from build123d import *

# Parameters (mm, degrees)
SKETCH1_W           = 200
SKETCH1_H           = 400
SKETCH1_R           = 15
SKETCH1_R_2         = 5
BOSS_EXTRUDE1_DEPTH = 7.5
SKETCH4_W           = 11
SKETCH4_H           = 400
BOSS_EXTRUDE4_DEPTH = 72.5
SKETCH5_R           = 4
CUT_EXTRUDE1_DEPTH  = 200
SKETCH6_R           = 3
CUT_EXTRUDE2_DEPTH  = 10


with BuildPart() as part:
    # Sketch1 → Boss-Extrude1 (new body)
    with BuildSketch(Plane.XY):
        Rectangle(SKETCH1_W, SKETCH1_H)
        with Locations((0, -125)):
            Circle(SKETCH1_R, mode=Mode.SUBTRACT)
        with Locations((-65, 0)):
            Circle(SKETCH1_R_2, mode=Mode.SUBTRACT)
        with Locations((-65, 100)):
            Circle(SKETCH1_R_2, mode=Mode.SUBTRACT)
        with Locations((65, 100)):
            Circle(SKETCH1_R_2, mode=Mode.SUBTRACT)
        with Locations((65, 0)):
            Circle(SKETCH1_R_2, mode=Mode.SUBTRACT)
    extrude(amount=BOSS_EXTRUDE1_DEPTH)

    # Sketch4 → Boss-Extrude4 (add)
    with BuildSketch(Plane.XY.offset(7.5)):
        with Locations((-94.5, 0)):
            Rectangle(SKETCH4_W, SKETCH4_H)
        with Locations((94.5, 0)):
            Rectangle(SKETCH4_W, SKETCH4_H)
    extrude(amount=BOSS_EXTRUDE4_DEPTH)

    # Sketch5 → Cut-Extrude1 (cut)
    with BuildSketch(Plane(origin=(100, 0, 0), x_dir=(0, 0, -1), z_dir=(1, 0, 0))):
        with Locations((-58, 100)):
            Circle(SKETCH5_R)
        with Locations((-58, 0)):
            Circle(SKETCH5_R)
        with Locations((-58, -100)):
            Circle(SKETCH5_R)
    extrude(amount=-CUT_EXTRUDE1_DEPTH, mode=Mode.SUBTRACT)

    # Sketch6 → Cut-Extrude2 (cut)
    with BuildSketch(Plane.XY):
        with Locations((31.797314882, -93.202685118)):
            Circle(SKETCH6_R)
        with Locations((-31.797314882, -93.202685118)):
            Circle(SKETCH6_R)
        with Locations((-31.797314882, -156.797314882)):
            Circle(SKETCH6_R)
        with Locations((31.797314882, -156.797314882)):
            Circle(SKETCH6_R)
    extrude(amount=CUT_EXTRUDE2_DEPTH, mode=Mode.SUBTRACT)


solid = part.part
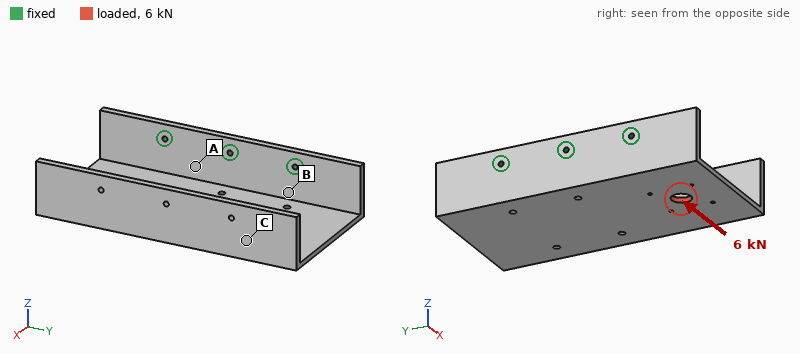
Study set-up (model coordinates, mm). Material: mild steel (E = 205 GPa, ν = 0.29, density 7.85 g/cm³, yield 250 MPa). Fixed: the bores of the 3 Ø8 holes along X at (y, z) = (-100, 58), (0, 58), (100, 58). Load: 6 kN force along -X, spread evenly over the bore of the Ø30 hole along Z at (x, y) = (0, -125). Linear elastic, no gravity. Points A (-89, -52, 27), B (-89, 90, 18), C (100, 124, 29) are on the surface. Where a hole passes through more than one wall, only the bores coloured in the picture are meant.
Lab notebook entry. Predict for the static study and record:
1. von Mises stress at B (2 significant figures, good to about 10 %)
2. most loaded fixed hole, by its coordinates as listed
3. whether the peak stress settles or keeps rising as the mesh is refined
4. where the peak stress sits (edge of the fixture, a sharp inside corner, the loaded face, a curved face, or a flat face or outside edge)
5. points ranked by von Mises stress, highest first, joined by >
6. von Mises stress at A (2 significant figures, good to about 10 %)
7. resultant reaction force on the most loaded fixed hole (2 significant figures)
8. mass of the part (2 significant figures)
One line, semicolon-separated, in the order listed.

24 MPa; (-100, 58); keeps rising; edge of the fixture; A > B > C; 39 MPa; 5.5 kN; 9.6 kg
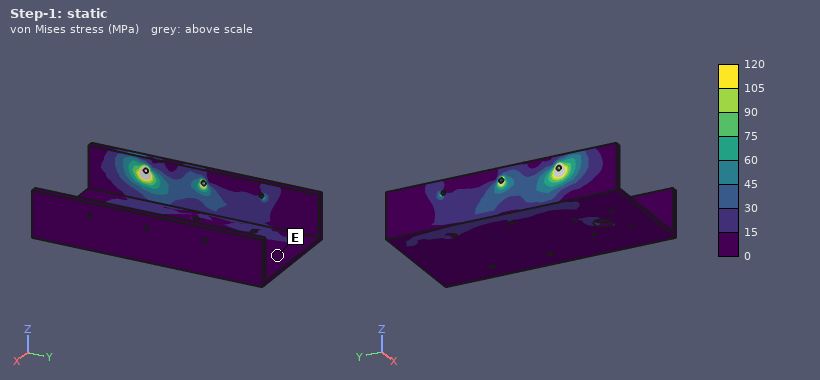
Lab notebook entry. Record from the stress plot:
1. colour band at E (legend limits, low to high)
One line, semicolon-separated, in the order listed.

0 to 15 MPa
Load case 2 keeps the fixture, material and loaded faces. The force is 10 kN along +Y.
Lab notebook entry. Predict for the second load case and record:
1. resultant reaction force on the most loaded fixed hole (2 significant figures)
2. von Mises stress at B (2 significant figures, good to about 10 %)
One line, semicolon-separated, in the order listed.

6.1 kN; 40 MPa
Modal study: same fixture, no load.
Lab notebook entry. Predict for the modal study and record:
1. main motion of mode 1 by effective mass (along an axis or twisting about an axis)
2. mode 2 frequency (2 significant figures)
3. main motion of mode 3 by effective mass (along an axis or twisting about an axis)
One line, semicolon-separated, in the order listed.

along Z; 150 Hz; along Y
